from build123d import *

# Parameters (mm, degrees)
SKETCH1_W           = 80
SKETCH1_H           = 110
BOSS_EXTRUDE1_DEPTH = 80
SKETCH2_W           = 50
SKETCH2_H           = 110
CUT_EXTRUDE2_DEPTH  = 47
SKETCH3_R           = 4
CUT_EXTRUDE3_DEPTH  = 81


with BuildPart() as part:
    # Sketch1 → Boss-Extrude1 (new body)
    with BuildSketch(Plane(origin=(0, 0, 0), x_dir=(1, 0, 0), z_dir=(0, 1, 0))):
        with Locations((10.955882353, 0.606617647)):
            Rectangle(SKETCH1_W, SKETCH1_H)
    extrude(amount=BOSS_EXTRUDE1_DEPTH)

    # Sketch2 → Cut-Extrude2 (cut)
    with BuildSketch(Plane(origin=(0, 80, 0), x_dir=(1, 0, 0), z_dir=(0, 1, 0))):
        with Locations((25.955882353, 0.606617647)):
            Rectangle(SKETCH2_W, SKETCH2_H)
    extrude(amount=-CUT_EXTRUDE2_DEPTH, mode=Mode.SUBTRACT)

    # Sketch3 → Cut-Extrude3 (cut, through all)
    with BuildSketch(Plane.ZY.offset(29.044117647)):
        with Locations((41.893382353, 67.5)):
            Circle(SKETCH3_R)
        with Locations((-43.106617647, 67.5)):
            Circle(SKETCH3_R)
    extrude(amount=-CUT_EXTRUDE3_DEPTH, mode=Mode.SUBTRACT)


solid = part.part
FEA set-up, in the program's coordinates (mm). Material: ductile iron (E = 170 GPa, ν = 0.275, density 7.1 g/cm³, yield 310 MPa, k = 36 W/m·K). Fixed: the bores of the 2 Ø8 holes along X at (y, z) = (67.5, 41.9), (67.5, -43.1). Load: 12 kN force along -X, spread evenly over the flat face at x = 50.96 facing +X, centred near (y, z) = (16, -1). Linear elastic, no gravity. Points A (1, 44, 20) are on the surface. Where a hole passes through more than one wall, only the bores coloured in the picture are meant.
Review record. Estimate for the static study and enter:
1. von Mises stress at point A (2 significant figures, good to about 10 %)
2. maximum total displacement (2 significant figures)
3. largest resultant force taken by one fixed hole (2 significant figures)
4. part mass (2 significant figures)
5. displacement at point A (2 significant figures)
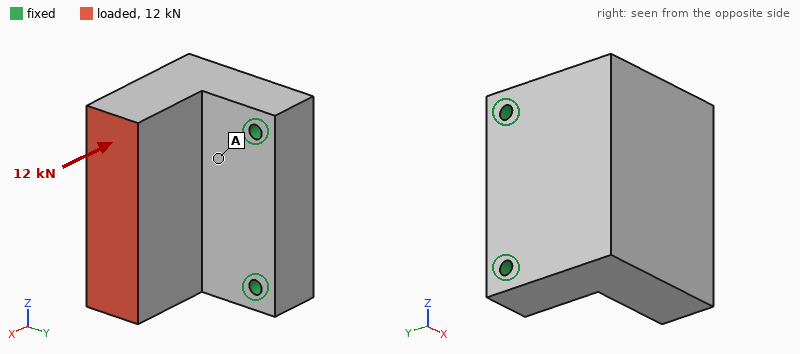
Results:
16 MPa
55 µm
6.0 kN
3.1 kg
14 µm
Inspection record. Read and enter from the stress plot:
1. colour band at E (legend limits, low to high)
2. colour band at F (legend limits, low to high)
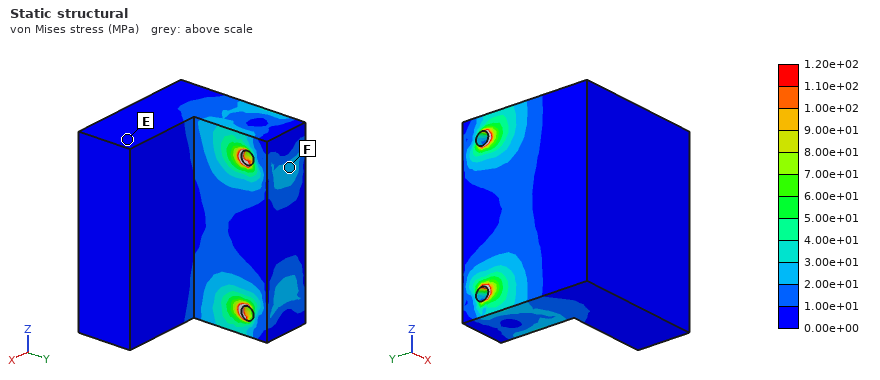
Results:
0.00e+00 to 1.00e+01 MPa
2.00e+01 to 3.00e+01 MPa
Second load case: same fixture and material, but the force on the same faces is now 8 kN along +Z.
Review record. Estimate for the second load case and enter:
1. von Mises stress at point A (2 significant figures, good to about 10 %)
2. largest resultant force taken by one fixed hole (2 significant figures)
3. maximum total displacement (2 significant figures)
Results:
20 MPa
8.3 kN
23 µm
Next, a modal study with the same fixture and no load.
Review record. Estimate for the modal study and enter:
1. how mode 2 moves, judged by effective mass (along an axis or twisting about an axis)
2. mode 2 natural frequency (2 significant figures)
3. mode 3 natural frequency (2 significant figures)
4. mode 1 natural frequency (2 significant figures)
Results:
along Z
3400 Hz
5200 Hz
1700 Hz
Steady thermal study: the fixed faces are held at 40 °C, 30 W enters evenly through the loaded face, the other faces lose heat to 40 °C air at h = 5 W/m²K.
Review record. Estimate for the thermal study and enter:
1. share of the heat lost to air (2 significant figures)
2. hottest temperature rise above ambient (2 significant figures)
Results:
8.1 %
26 K
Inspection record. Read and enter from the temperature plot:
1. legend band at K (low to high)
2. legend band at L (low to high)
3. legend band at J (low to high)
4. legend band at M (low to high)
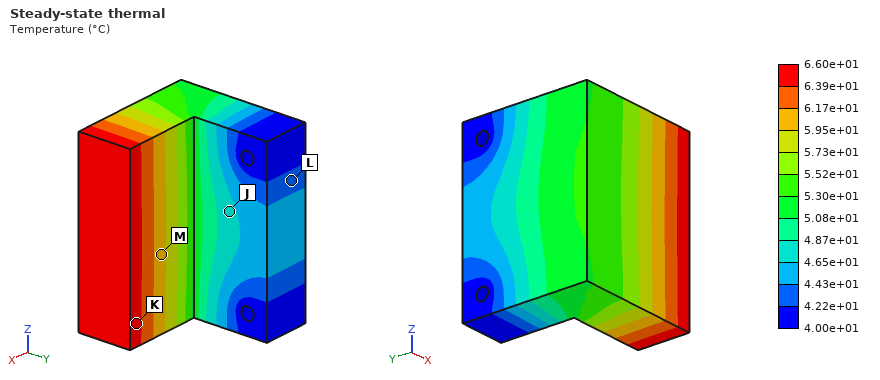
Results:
6.39e+01 to 6.60e+01 °C
4.22e+01 to 4.43e+01 °C
4.65e+01 to 4.87e+01 °C
5.95e+01 to 6.17e+01 °C
